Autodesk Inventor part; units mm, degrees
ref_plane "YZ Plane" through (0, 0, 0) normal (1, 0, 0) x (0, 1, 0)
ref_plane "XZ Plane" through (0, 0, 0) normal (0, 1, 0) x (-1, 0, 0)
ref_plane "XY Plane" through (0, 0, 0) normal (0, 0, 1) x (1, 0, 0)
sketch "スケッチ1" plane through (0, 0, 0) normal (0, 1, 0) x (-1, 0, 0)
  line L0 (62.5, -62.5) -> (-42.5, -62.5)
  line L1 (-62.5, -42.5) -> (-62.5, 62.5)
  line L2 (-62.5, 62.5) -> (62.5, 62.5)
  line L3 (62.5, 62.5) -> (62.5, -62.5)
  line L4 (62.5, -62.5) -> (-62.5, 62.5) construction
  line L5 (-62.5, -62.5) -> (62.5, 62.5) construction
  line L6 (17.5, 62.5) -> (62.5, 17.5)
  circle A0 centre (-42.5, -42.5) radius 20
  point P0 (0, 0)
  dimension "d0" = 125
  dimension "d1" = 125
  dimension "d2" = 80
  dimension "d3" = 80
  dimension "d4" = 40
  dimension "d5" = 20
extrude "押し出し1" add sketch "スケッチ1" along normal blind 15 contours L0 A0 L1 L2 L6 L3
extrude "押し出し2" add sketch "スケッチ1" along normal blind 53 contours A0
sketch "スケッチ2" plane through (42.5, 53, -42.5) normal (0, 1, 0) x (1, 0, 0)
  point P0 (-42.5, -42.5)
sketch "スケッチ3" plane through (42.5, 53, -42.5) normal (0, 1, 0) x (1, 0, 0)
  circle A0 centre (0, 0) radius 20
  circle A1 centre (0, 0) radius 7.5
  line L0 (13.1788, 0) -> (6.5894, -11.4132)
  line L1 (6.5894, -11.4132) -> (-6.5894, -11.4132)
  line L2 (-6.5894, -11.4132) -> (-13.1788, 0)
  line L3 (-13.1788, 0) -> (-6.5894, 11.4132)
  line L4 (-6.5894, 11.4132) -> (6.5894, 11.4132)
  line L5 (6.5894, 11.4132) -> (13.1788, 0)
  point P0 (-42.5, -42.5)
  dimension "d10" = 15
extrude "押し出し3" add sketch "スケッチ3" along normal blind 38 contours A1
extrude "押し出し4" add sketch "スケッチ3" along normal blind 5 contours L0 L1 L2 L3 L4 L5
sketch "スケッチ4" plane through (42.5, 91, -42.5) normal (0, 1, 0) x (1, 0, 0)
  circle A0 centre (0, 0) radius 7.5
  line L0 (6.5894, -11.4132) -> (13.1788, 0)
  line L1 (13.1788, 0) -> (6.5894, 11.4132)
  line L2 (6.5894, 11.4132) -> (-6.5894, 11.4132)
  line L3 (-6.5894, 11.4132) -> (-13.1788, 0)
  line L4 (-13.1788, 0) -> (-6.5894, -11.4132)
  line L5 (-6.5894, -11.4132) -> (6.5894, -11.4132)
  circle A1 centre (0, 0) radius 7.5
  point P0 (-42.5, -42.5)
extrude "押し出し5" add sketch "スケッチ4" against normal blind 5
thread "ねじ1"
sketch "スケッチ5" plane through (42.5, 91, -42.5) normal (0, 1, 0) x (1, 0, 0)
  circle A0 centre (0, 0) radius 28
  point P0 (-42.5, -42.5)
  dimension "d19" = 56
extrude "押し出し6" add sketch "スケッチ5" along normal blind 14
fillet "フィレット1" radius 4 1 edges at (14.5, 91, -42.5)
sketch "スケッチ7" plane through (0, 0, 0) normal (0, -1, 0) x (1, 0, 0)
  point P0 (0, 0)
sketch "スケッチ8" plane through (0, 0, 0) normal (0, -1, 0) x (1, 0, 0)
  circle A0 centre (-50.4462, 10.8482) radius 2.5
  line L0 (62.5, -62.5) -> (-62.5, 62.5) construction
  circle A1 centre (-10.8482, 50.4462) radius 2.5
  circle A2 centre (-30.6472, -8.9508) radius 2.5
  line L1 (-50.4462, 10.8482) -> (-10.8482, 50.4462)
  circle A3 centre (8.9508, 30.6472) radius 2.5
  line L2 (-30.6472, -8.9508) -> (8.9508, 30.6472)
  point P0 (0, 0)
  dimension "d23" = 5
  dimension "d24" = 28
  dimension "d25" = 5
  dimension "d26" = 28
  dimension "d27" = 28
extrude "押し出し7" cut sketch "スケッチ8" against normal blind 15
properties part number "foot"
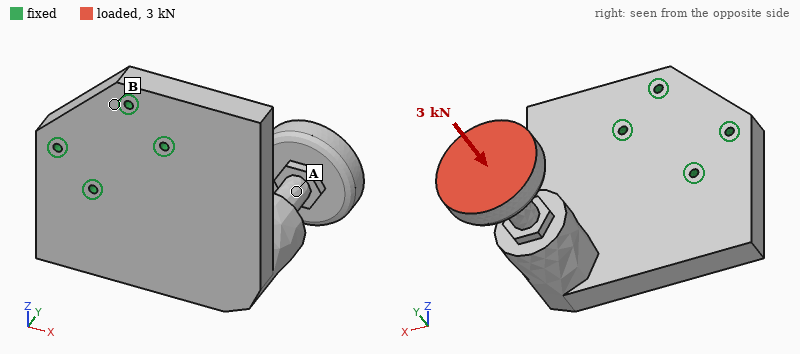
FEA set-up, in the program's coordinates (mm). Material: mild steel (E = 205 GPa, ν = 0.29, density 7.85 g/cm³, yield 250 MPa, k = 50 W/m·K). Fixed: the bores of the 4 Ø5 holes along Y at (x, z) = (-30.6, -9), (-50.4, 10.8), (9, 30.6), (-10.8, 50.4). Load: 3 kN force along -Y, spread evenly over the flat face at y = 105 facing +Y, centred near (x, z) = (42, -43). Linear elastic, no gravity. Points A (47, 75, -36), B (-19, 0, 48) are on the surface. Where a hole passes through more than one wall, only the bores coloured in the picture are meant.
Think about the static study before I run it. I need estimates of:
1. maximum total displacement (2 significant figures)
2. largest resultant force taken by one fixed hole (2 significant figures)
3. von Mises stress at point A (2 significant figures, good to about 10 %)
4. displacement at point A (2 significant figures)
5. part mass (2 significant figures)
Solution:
0.19 mm
3.5 kN
17 MPa
0.13 mm
2.4 kg
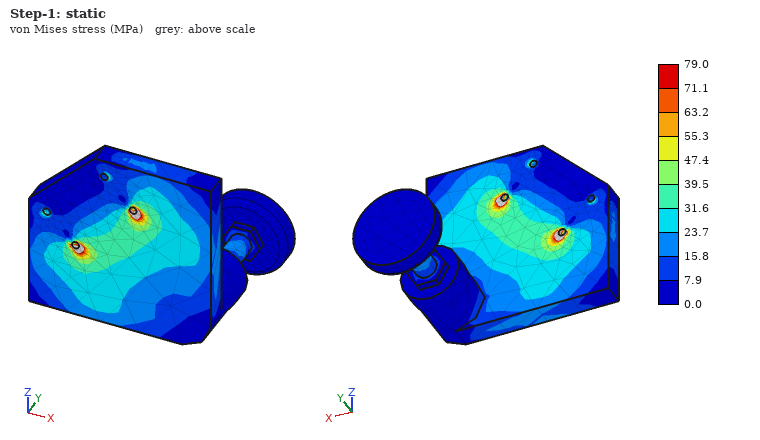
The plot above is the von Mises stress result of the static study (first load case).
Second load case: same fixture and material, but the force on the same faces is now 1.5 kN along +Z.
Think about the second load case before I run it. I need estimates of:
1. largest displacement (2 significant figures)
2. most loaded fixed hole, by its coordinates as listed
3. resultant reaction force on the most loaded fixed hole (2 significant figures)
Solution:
0.32 mm
(-30.6, -9)
3.0 kN
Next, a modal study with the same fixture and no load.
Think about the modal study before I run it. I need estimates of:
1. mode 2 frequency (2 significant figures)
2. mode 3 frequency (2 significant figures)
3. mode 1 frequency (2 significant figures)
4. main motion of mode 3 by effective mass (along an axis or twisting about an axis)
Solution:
830 Hz
1400 Hz
610 Hz
along Y
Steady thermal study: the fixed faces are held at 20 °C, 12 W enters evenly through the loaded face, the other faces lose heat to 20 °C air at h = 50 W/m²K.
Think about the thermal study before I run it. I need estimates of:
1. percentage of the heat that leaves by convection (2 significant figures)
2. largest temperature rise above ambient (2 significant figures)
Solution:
84 %
28 K
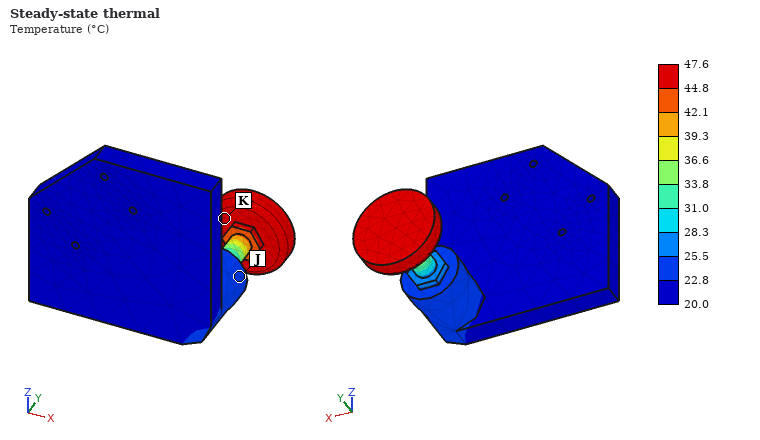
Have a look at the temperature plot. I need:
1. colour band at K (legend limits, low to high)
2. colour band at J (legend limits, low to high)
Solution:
44.8 to 47.6 °C
22.8 to 25.5 °C
